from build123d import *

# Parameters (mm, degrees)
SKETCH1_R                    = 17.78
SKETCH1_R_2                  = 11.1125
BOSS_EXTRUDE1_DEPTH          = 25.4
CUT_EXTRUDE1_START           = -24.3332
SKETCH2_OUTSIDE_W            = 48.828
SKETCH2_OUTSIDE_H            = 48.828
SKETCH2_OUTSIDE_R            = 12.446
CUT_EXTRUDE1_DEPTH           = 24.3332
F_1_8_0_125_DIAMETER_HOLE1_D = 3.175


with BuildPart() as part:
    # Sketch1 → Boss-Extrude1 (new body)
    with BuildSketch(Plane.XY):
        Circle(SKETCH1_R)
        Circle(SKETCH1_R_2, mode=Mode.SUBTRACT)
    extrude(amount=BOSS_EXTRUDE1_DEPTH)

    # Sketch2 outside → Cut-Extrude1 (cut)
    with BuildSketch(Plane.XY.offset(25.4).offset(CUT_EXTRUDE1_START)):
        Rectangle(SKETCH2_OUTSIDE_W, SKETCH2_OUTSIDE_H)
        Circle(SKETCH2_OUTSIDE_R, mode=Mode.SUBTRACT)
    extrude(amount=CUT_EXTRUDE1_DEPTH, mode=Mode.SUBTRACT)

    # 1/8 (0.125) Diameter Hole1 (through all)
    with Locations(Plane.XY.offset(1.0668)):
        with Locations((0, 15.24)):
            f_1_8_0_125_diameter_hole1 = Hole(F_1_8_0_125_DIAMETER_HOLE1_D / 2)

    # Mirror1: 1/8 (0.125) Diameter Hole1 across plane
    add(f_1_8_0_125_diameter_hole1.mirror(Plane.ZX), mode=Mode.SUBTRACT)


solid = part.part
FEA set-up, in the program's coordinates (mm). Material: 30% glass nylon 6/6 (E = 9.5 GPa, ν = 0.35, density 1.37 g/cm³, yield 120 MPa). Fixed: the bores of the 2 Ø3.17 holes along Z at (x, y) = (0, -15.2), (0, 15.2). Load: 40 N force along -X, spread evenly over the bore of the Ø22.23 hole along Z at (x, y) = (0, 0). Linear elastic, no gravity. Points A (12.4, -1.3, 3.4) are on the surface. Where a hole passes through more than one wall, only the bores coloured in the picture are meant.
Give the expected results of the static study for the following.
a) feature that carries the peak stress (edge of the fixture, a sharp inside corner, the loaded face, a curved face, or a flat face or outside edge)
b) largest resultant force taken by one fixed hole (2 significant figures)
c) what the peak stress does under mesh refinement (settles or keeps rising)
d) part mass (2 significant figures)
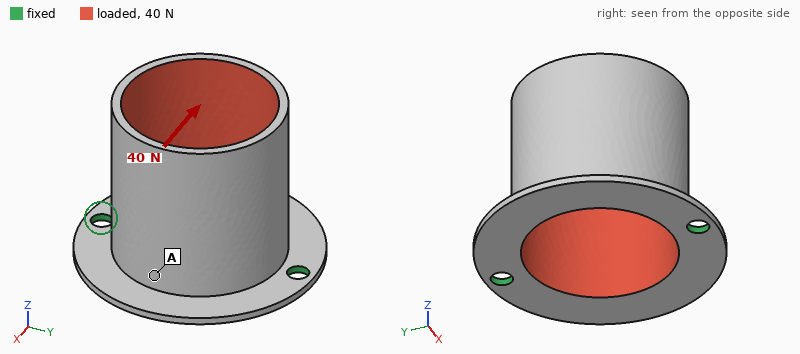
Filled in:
edge of the fixture
20 N
keeps rising
4.2 g
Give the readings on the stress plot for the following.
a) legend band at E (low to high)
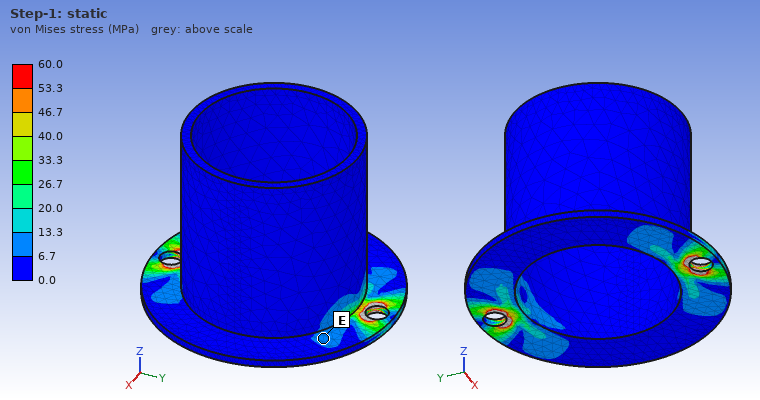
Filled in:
6.7 to 13.3 MPa
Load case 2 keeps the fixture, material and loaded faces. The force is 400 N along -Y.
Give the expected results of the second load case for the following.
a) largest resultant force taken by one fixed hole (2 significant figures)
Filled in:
270 N
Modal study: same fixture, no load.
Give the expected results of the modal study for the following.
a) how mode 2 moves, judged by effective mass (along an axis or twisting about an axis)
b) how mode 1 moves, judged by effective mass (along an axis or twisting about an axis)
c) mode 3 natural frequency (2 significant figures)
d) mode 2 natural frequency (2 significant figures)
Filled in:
along Z
along X
3600 Hz
3200 Hz
